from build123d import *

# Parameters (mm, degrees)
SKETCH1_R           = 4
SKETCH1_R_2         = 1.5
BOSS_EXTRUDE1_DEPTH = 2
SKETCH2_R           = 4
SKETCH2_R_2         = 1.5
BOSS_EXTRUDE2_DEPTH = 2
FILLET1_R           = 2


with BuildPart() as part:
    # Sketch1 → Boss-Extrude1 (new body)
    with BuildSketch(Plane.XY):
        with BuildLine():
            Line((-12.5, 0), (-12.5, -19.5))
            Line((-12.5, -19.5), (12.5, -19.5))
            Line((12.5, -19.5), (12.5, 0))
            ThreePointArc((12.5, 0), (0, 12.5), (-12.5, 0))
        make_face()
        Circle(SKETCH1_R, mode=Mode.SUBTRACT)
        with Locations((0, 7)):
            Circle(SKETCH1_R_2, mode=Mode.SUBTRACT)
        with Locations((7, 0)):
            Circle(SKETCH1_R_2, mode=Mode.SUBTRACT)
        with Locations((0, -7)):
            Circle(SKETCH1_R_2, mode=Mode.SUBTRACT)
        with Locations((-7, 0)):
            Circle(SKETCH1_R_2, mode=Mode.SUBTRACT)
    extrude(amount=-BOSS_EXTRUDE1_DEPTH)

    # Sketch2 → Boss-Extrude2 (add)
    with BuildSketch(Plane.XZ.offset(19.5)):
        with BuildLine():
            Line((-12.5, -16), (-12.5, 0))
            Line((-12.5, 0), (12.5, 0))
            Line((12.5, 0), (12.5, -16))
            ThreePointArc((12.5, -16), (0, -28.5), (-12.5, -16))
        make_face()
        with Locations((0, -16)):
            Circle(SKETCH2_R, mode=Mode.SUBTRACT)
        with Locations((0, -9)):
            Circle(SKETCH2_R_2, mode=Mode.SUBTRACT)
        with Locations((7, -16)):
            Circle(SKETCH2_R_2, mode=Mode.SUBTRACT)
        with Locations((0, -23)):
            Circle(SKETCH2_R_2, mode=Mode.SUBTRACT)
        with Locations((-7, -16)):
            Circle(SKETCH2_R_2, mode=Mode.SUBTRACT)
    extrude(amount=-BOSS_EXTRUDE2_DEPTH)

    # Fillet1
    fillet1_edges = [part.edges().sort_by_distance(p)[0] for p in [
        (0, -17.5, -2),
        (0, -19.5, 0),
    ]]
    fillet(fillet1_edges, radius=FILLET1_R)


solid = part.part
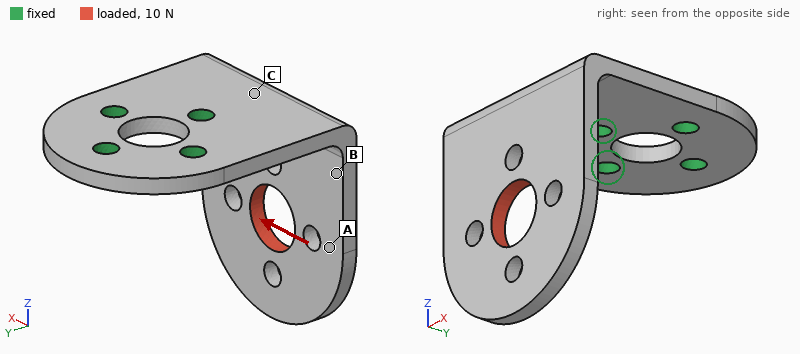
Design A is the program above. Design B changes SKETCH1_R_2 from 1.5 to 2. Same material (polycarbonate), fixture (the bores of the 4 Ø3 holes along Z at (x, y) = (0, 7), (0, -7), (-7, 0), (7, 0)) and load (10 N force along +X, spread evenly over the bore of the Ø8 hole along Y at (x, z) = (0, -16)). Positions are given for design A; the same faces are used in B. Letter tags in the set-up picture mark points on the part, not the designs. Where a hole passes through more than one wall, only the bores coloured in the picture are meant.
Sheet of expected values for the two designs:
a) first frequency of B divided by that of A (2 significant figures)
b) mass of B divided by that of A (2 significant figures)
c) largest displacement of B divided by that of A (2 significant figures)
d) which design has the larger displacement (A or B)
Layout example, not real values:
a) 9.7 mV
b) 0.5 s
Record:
a) 1.0
b) 0.98
c) 0.90
d) A
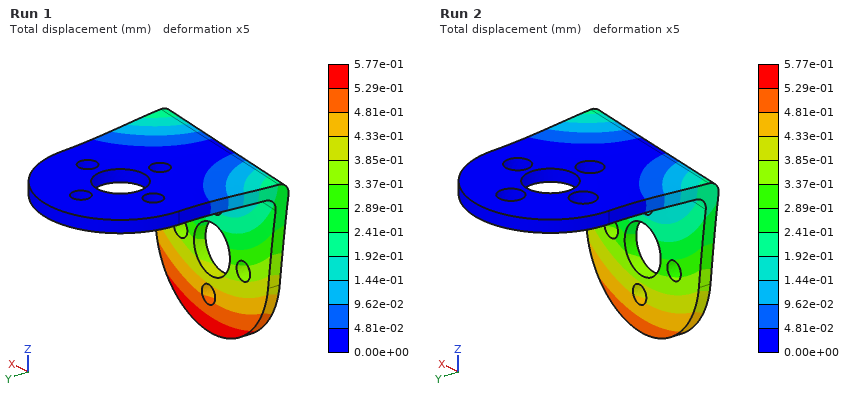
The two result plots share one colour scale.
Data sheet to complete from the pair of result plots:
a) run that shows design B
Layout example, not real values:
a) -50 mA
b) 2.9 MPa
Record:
a) Run 2
